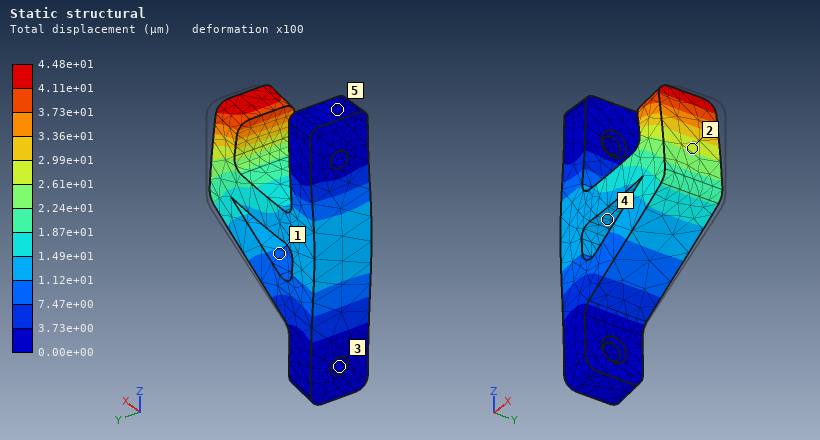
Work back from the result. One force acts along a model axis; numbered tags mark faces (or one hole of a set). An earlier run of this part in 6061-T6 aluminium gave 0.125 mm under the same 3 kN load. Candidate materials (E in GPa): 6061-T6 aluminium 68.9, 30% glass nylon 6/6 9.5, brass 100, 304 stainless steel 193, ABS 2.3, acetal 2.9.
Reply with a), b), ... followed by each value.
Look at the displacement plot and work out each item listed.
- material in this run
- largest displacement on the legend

a) 304 stainless steel
b) 4.48e+01 µm
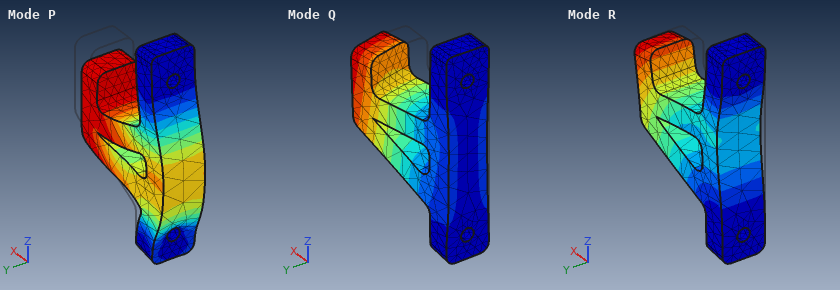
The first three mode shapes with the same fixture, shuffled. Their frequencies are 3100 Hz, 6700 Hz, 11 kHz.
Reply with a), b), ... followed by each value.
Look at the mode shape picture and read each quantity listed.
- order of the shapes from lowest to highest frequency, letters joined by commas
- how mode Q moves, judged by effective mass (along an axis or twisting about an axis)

a) Q, R, P
b) along Y
